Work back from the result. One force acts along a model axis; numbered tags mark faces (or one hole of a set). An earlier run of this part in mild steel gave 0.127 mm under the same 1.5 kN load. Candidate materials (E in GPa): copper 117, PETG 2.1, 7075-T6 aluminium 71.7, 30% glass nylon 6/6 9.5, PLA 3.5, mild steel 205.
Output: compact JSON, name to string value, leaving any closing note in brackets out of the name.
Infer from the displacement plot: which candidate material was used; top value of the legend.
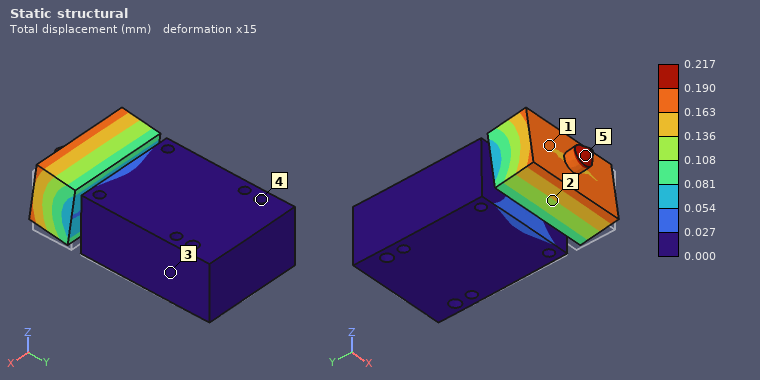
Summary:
{"which candidate material was used": "copper", "top value of the legend": "0.217 mm"}
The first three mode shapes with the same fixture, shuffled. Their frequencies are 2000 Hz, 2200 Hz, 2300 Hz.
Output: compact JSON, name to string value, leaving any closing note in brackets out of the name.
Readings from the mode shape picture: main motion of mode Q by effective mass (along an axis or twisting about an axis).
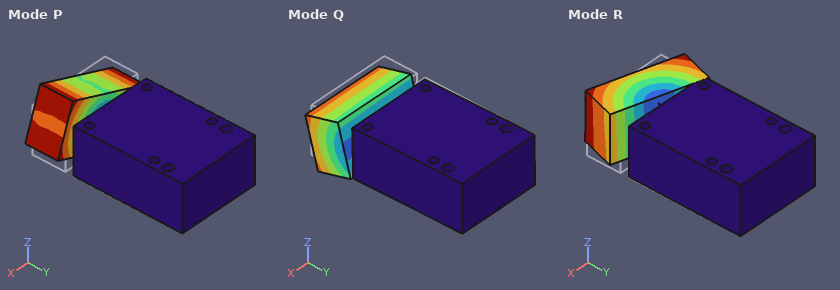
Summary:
{"main motion of mode Q by effective mass": "along Z"}
